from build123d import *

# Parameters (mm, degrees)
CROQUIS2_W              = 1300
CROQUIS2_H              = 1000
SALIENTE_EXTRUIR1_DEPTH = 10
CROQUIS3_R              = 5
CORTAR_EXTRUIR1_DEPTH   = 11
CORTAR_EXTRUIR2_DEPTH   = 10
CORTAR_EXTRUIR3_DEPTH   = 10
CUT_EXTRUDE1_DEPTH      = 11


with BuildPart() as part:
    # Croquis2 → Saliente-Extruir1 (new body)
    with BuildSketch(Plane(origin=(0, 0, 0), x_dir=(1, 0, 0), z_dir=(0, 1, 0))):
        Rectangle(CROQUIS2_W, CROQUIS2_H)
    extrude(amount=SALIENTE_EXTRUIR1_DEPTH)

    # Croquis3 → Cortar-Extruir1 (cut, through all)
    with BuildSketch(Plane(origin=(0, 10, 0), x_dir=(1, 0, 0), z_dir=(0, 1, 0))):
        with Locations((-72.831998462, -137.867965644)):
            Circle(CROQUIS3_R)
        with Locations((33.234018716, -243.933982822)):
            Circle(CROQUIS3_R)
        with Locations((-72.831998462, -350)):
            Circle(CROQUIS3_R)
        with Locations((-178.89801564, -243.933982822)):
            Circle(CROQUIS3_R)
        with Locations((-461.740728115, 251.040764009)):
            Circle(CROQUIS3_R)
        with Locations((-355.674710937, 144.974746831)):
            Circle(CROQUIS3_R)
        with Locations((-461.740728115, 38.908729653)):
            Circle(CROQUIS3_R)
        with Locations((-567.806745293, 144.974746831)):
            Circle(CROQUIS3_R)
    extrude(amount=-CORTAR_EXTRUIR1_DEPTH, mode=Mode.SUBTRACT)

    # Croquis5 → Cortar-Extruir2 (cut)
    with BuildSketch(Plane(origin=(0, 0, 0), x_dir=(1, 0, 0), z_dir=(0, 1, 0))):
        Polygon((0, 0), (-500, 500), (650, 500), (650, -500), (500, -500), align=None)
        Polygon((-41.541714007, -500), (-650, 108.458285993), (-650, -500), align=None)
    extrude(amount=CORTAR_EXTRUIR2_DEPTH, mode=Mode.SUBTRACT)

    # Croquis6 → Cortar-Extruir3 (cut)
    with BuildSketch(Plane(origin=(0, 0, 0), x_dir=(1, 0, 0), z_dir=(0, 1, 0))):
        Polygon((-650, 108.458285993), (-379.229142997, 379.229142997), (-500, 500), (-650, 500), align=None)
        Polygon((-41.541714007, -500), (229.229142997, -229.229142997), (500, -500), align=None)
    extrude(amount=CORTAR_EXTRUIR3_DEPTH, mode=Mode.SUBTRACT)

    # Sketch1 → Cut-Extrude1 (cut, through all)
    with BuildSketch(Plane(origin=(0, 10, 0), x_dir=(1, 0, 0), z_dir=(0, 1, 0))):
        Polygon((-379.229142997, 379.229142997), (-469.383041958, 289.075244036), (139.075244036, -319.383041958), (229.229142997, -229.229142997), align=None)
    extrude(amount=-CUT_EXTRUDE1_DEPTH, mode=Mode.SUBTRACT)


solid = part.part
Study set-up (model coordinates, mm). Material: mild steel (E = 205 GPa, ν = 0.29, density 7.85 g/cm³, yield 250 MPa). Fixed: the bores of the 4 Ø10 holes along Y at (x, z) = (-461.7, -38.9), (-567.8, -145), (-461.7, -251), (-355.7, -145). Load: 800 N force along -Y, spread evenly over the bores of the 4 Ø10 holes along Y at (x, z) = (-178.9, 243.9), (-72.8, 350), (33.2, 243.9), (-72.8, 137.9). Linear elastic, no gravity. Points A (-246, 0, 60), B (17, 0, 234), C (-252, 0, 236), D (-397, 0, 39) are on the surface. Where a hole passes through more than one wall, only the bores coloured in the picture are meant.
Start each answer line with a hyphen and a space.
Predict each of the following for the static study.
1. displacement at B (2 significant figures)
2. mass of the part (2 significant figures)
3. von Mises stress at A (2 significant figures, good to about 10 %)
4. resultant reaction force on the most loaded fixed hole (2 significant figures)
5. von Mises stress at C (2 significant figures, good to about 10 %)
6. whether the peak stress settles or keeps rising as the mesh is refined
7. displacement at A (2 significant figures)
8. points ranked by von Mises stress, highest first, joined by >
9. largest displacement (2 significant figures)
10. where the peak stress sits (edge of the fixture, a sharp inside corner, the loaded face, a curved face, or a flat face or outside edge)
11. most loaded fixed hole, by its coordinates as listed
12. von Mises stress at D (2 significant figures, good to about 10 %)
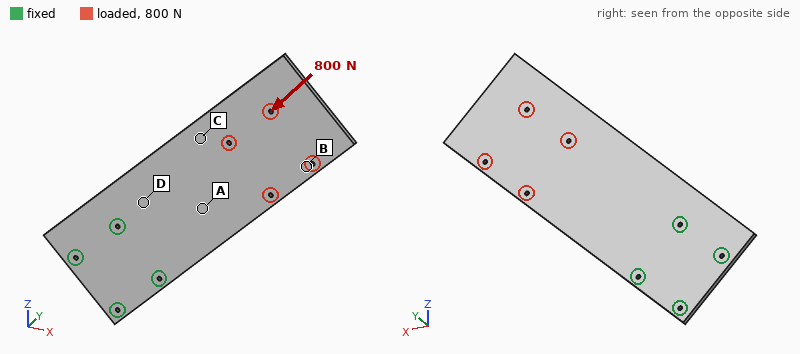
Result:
- 8.2 mm
- 17 kg
- 47 MPa
- 1.2 kN
- 25 MPa
- keeps rising
- 2.0 mm
- D > A > C > B
- 11 mm
- edge of the fixture
- (-461.7, -38.9)
- 64 MPa
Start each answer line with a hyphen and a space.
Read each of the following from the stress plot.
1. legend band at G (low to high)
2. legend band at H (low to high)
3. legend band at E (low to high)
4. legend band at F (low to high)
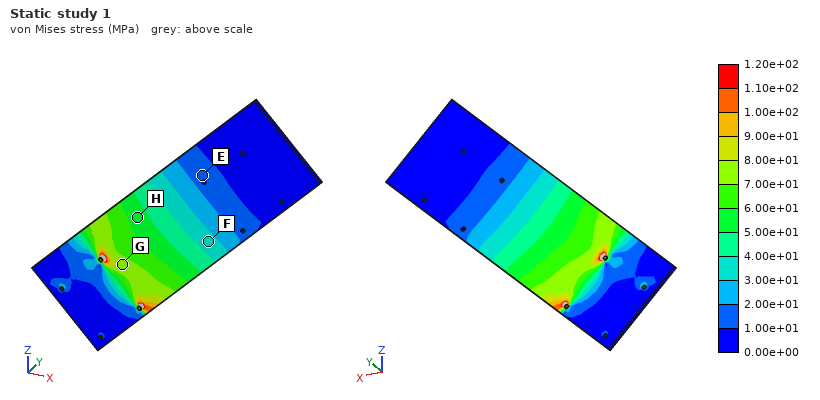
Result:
- 7.00e+01 to 8.00e+01 MPa
- 5.00e+01 to 6.00e+01 MPa
- 1.00e+01 to 2.00e+01 MPa
- 3.00e+01 to 4.00e+01 MPa
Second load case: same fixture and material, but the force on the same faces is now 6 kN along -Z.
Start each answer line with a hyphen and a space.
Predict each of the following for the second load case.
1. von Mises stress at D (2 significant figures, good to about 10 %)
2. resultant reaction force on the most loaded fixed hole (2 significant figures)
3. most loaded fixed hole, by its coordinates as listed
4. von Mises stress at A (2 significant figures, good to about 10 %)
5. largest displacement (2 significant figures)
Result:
- 6.1 MPa
- 12 kN
- (-355.7, -145)
- 6.4 MPa
- 0.14 mm
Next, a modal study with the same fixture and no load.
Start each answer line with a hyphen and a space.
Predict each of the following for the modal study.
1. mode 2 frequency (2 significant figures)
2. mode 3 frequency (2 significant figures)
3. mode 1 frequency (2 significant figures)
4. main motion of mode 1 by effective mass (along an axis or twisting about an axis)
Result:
- 98 Hz
- 110 Hz
- 18 Hz
- along Y
